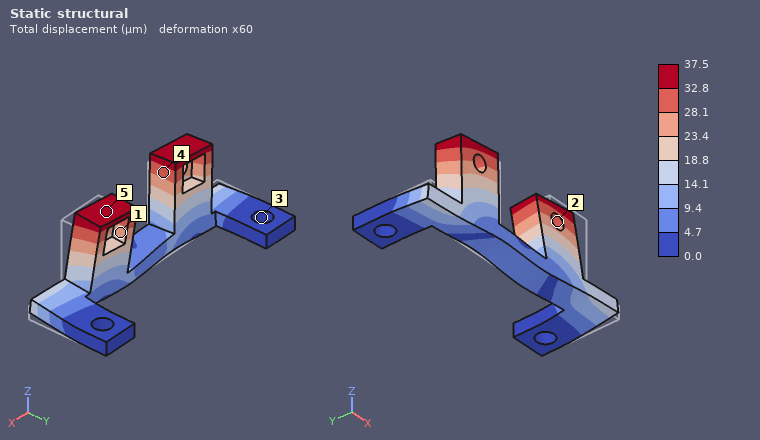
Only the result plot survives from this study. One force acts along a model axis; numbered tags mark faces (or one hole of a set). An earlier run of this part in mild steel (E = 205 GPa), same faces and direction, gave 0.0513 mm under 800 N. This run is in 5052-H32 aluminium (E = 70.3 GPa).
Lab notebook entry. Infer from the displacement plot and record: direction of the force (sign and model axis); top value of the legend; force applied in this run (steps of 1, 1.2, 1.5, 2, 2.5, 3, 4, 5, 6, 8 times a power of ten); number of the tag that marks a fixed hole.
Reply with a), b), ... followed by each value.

a) -X
b) 37.5 µm
c) 200 N
d) 3
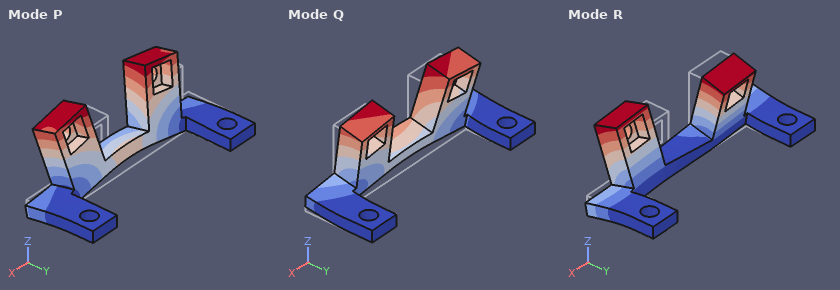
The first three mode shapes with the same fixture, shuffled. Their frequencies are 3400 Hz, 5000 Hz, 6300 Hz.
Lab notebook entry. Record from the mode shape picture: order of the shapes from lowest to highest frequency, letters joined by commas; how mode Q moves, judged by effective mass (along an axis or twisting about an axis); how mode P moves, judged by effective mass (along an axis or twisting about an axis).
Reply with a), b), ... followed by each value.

a) Q, P, R
b) along Z
c) along Y
